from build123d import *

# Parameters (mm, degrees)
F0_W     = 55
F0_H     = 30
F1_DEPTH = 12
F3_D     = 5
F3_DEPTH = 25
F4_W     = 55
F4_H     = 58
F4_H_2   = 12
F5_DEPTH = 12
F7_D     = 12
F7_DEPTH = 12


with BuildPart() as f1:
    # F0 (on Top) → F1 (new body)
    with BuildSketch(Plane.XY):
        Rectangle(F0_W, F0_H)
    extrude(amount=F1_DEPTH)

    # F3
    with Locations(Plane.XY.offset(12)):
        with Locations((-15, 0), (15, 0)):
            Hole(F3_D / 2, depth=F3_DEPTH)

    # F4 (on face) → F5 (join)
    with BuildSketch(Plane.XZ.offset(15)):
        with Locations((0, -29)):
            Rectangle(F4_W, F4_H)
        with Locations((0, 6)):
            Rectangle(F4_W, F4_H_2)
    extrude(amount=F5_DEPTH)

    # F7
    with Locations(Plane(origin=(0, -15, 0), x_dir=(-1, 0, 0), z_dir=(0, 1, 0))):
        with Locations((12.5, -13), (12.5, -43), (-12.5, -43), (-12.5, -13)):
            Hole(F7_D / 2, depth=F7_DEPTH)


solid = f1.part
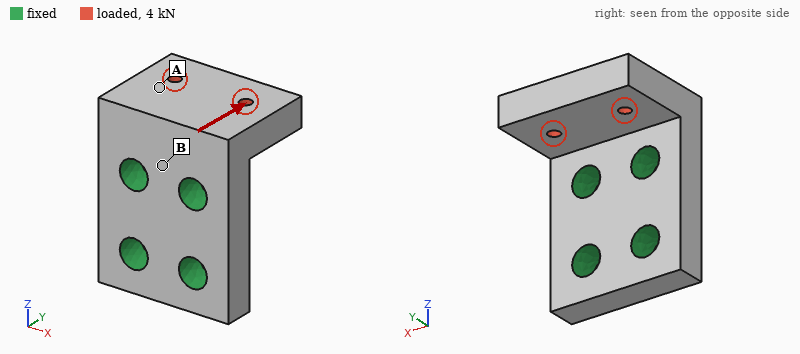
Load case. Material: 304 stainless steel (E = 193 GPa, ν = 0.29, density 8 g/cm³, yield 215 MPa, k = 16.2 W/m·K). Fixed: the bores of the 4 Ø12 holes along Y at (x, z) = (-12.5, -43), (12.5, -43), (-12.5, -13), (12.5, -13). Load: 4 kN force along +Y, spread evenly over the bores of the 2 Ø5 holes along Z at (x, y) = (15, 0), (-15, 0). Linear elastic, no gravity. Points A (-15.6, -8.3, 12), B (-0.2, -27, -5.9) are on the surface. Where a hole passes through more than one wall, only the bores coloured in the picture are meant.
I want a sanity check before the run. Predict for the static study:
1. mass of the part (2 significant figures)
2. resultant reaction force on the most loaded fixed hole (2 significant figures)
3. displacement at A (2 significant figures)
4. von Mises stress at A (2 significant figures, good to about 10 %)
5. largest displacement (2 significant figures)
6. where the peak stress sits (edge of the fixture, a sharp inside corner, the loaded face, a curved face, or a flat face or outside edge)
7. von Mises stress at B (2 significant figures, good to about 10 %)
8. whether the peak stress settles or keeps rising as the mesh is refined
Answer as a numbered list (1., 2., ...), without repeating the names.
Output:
1. 480 g
2. 2.1 kN
3. 8.3 µm
4. 9.2 MPa
5. 15 µm
6. edge of the fixture
7. 20 MPa
8. keeps rising
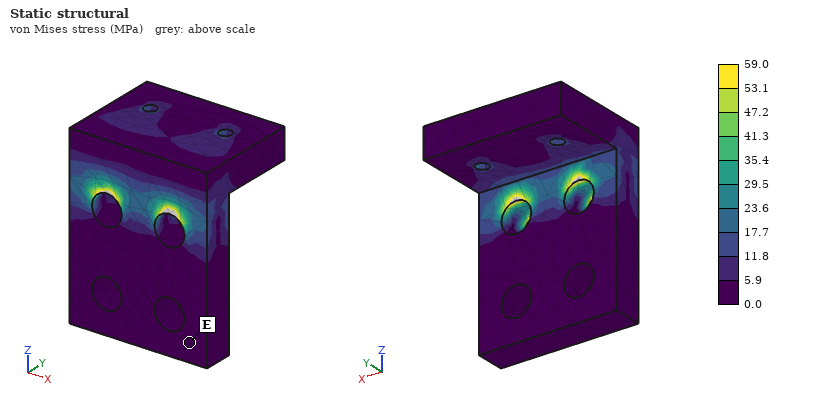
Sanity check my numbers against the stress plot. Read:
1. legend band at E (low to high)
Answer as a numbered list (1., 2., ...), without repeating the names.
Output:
1. 0.0 to 5.9 MPa
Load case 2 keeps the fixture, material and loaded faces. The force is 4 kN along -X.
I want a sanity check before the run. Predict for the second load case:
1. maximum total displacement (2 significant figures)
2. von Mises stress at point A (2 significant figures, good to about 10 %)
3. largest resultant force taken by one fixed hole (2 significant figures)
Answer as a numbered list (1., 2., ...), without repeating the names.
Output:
1. 13 µm
2. 4.9 MPa
3. 3.4 kN
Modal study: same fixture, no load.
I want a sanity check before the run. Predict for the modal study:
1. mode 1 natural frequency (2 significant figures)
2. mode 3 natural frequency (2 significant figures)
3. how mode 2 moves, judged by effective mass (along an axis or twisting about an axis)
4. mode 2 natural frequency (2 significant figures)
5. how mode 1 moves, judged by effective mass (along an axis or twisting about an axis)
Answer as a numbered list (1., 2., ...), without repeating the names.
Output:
1. 4500 Hz
2. 11 kHz
3. along X
4. 7500 Hz
5. along Z
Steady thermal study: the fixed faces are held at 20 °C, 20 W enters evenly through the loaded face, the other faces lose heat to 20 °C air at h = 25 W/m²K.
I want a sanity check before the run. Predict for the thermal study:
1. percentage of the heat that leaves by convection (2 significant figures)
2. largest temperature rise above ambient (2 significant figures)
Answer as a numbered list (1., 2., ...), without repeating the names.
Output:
1. 28 %
2. 54 K
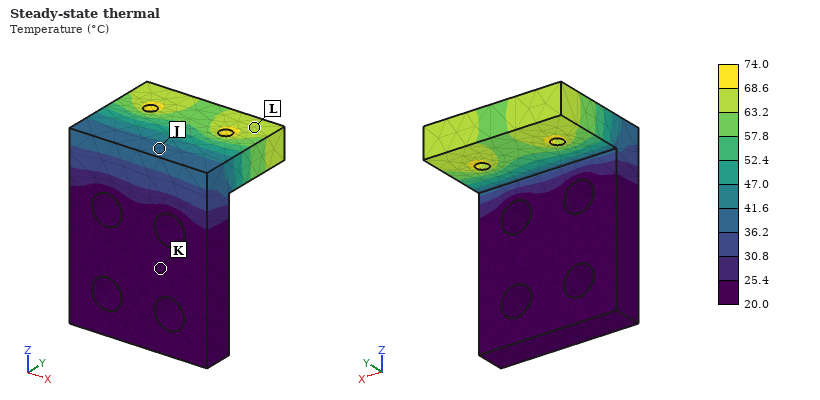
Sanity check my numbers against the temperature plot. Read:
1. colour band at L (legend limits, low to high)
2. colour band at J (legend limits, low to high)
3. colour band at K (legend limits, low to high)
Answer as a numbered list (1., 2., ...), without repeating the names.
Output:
1. 63.2 to 68.6 °C
2. 36.2 to 41.6 °C
3. 20.0 to 25.4 °C
